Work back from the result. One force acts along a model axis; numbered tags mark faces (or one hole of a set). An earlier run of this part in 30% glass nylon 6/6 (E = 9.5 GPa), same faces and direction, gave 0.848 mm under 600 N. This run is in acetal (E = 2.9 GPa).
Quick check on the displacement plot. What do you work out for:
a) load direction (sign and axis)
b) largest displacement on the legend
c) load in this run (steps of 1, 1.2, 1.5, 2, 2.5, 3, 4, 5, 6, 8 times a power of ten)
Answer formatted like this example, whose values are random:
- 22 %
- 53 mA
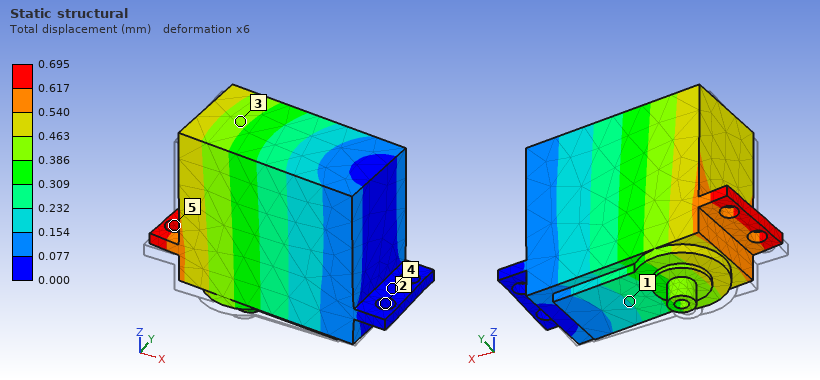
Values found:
- +Y
- 0.695 mm
- 150 N
